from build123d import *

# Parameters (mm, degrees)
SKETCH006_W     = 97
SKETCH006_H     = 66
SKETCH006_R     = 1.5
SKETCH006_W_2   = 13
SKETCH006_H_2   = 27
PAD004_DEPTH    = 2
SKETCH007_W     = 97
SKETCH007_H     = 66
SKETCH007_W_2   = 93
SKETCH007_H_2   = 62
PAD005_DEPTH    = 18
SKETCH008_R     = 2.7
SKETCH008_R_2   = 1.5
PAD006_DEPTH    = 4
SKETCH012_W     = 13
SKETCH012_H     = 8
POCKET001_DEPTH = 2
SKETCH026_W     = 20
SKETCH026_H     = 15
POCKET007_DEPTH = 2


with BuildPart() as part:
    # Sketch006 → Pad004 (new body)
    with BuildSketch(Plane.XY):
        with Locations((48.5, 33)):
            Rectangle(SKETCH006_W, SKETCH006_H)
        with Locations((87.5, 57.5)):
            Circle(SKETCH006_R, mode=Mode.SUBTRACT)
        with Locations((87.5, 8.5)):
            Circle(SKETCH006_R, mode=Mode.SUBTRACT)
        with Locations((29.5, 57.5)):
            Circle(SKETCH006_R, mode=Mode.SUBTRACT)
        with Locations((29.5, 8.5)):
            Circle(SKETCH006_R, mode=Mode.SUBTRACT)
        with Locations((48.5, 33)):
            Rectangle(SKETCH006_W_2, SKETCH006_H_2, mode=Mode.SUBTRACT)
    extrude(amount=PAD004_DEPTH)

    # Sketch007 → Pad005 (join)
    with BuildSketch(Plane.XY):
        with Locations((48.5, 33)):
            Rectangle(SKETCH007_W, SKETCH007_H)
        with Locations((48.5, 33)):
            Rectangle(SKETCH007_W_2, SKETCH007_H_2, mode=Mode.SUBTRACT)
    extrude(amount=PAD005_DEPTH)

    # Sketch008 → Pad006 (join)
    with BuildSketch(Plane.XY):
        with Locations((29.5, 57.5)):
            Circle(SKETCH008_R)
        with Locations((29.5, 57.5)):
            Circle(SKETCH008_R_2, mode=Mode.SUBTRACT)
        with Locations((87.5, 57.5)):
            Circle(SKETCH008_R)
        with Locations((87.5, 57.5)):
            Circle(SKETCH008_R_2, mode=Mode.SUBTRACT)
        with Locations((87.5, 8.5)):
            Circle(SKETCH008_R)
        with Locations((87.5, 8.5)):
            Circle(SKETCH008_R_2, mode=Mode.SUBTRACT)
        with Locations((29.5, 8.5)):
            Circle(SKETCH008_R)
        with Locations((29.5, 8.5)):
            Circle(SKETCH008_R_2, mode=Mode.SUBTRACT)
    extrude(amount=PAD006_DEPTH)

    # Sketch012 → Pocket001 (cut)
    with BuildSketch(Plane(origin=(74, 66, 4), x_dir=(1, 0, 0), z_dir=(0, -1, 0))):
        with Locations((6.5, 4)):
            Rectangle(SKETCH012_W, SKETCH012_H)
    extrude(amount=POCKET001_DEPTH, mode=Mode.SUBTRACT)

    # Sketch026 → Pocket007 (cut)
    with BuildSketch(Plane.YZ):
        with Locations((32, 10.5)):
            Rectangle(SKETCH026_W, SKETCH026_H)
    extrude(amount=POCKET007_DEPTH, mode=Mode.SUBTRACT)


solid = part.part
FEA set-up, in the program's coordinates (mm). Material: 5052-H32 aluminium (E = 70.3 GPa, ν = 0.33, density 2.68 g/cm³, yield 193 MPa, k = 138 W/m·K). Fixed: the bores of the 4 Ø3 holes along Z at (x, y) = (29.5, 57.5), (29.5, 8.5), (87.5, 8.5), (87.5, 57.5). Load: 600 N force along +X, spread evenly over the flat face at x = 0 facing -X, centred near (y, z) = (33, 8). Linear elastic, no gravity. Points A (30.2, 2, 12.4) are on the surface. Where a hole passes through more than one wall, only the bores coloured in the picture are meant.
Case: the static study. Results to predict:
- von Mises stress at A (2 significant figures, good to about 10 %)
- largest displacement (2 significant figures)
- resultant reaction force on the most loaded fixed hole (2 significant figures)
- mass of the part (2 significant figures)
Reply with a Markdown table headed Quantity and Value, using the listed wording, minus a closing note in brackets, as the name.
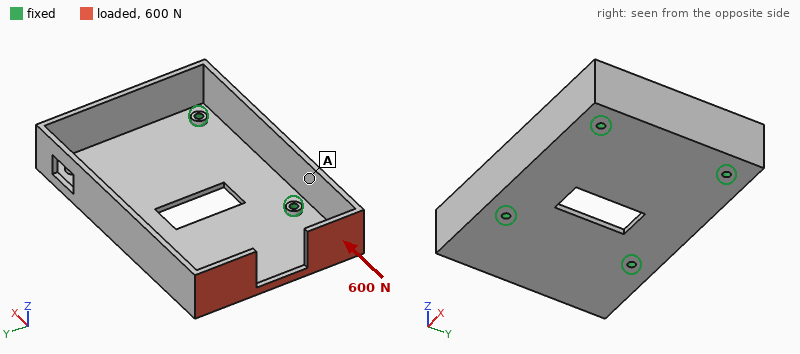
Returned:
| Quantity | Value |
|---|---|
| von Mises stress at A | 6.3 MPa |
| largest displacement | 0.16 mm |
| resultant reaction force on the most loaded fixed hole | 210 N |
| mass of the part | 58 g |
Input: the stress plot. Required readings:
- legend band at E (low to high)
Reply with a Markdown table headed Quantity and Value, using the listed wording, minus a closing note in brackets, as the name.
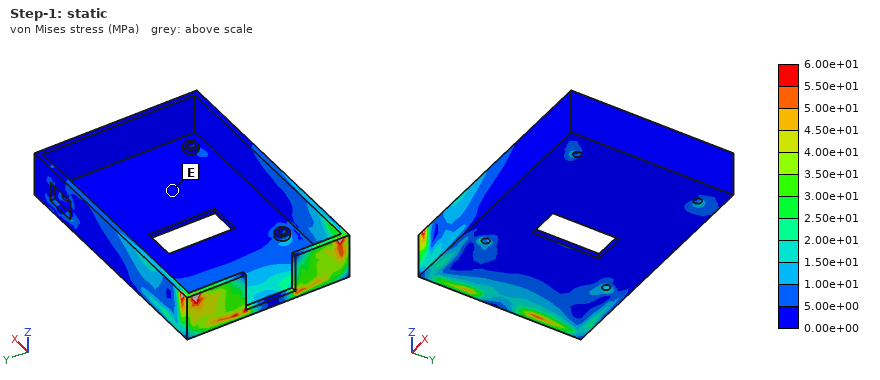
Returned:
| Quantity | Value |
|---|---|
| legend band at E | 0.00e+00 to 5.00e+00 MPa |
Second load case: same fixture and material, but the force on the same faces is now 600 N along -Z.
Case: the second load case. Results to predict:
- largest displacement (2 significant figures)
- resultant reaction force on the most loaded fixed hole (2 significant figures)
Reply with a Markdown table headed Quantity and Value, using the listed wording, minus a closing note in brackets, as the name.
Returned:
| Quantity | Value |
|---|---|
| largest displacement | 0.45 mm |
| resultant reaction force on the most loaded fixed hole | 510 N |
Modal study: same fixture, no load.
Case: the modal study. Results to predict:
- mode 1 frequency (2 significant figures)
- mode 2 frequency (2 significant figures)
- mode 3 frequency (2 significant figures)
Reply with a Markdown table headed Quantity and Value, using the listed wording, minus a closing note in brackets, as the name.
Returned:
| Quantity | Value |
|---|---|
| mode 1 frequency | 2100 Hz |
| mode 2 frequency | 2900 Hz |
| mode 3 frequency | 3500 Hz |
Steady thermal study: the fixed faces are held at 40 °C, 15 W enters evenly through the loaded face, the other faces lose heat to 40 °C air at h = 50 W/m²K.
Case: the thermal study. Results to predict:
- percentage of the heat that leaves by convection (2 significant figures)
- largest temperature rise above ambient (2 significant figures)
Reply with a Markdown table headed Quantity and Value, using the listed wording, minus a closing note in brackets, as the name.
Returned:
| Quantity | Value |
|---|---|
| percentage of the heat that leaves by convection | 33 % |
| largest temperature rise above ambient | 23 K |
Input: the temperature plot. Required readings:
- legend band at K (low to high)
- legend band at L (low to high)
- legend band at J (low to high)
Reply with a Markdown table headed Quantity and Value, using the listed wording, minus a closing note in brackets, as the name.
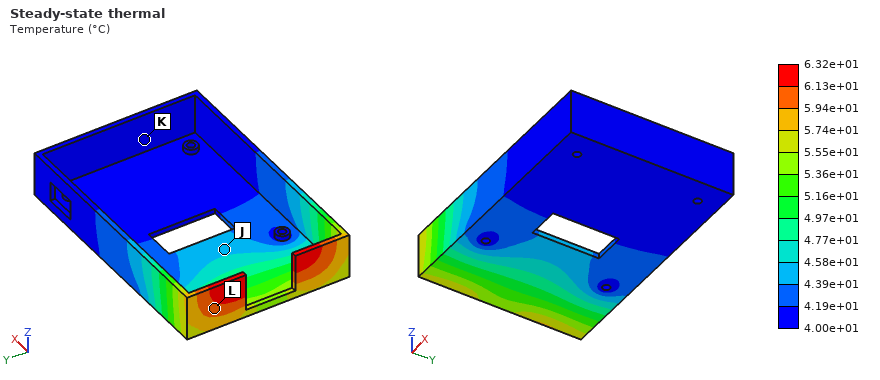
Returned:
| Quantity | Value |
|---|---|
| legend band at K | 4.00e+01 to 4.19e+01 °C |
| legend band at L | 5.94e+01 to 6.13e+01 °C |
| legend band at J | 4.39e+01 to 4.58e+01 °C |
